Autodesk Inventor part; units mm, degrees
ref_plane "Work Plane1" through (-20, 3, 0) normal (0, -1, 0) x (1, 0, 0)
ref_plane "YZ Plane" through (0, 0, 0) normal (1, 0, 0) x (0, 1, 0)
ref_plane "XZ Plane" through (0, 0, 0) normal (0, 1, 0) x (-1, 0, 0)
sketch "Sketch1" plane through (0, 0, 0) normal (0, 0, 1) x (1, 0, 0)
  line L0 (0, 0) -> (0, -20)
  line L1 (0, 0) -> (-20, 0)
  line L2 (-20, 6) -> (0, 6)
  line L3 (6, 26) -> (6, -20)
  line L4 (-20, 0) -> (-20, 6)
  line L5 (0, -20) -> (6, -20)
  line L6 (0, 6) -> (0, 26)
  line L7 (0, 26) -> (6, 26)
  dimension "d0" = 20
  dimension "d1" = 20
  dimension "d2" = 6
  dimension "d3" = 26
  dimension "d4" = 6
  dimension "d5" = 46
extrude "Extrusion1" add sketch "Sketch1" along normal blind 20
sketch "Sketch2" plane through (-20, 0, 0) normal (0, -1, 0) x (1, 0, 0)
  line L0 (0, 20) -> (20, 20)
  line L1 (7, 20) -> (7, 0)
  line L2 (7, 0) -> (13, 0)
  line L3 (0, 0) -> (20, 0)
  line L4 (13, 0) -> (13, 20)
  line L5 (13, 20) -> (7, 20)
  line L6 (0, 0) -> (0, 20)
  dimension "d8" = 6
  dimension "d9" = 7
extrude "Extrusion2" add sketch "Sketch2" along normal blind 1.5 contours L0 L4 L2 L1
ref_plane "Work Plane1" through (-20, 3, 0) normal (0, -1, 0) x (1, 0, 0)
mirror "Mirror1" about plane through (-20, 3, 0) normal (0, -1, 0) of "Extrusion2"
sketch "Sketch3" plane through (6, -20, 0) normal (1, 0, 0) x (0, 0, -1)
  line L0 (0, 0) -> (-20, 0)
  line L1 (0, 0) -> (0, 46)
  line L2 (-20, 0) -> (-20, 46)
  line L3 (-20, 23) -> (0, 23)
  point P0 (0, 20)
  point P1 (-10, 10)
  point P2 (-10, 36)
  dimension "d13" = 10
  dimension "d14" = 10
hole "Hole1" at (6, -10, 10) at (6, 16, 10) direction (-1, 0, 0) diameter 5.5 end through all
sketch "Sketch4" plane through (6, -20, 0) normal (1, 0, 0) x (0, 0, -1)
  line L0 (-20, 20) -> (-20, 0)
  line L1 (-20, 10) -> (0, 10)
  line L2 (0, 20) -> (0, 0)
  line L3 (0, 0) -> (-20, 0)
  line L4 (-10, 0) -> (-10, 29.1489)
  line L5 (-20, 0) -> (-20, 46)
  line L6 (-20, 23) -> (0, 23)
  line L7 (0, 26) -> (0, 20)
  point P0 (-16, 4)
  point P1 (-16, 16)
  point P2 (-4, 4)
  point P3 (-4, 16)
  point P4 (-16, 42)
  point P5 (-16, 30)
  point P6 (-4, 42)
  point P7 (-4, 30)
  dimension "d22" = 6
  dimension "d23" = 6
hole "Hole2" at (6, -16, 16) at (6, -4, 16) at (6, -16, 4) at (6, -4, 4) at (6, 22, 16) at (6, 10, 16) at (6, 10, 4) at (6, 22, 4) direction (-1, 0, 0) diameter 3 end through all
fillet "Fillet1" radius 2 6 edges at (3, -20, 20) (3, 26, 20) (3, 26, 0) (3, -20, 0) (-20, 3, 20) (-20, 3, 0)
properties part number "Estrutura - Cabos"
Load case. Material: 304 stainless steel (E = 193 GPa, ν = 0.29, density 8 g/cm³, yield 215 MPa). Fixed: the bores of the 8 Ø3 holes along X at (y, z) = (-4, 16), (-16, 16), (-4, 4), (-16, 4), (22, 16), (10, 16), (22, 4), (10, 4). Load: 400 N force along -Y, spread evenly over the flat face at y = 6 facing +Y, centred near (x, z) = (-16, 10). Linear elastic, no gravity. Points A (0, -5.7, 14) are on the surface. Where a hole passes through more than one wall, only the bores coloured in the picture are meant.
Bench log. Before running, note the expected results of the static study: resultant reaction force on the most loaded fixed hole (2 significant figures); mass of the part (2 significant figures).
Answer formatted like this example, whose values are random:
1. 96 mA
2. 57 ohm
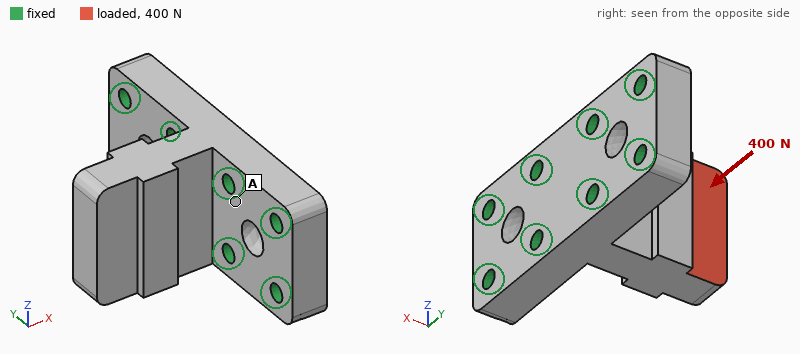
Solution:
1. 340 N
2. 61 g
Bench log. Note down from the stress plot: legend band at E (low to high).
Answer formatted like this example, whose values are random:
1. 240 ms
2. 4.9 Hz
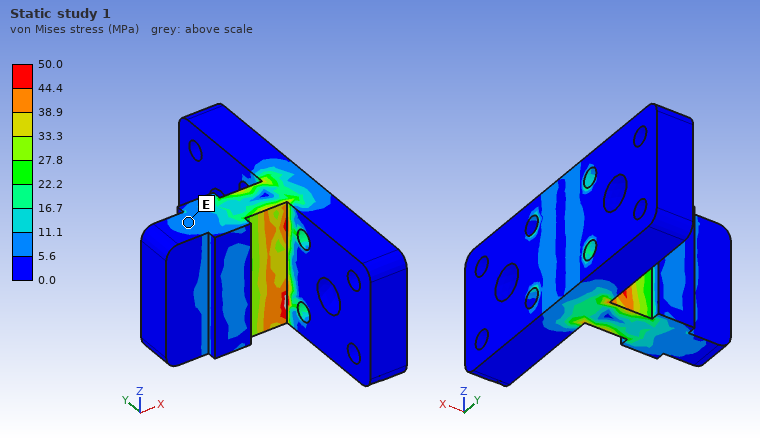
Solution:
1. 5.6 to 11.1 MPa
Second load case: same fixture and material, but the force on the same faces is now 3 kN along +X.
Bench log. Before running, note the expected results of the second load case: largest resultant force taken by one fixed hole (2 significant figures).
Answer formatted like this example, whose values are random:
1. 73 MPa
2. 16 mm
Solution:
1. 1.2 kN
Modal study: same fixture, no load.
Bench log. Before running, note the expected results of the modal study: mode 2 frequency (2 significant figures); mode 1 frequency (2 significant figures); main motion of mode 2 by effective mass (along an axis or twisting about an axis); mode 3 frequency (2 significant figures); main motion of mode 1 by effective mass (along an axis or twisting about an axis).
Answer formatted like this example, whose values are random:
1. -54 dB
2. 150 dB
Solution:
1. 16 kHz
2. 9200 Hz
3. along Z
4. 22 kHz
5. along Y
